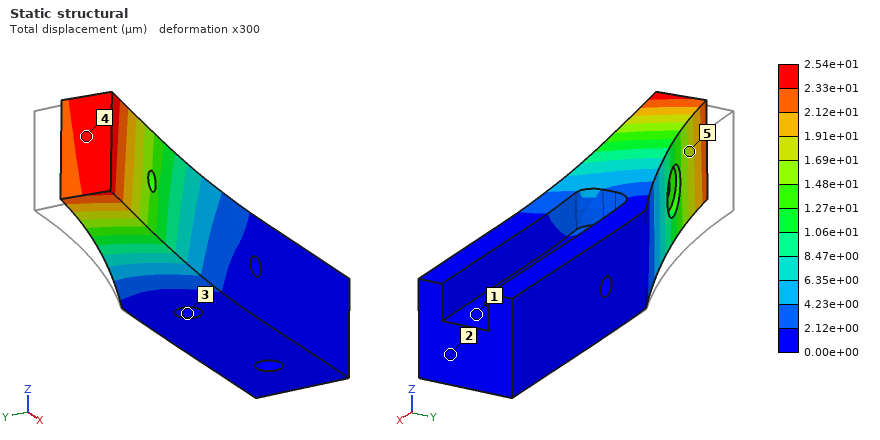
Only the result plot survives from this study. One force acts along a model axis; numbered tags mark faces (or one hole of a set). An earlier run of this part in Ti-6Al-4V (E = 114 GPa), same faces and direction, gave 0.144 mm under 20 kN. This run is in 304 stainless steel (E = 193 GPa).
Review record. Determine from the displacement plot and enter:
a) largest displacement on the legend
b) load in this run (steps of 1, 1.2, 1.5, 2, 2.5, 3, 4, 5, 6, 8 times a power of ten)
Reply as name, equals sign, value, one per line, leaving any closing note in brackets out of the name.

largest displacement on the legend = 2.54e+01 µm
load in this run = 6 kN
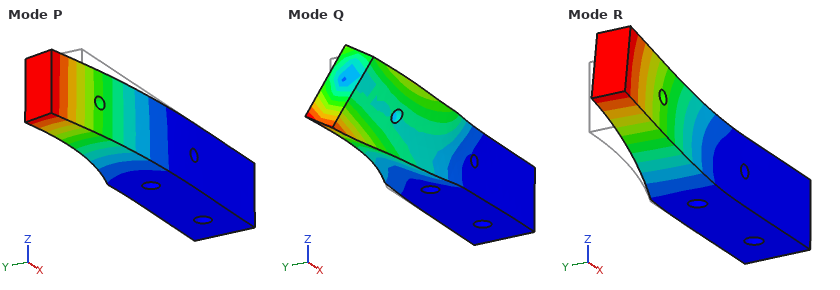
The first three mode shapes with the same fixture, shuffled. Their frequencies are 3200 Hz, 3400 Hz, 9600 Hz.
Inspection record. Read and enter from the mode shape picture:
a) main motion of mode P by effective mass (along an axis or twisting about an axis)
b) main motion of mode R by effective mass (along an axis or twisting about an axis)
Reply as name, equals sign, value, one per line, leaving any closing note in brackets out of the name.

main motion of mode P by effective mass = along Y
main motion of mode R by effective mass = along Z
